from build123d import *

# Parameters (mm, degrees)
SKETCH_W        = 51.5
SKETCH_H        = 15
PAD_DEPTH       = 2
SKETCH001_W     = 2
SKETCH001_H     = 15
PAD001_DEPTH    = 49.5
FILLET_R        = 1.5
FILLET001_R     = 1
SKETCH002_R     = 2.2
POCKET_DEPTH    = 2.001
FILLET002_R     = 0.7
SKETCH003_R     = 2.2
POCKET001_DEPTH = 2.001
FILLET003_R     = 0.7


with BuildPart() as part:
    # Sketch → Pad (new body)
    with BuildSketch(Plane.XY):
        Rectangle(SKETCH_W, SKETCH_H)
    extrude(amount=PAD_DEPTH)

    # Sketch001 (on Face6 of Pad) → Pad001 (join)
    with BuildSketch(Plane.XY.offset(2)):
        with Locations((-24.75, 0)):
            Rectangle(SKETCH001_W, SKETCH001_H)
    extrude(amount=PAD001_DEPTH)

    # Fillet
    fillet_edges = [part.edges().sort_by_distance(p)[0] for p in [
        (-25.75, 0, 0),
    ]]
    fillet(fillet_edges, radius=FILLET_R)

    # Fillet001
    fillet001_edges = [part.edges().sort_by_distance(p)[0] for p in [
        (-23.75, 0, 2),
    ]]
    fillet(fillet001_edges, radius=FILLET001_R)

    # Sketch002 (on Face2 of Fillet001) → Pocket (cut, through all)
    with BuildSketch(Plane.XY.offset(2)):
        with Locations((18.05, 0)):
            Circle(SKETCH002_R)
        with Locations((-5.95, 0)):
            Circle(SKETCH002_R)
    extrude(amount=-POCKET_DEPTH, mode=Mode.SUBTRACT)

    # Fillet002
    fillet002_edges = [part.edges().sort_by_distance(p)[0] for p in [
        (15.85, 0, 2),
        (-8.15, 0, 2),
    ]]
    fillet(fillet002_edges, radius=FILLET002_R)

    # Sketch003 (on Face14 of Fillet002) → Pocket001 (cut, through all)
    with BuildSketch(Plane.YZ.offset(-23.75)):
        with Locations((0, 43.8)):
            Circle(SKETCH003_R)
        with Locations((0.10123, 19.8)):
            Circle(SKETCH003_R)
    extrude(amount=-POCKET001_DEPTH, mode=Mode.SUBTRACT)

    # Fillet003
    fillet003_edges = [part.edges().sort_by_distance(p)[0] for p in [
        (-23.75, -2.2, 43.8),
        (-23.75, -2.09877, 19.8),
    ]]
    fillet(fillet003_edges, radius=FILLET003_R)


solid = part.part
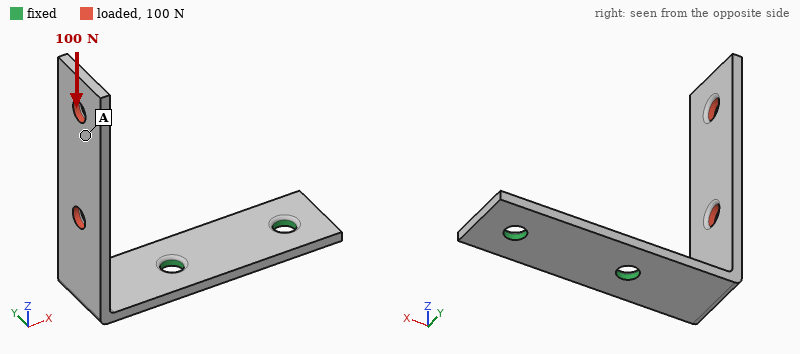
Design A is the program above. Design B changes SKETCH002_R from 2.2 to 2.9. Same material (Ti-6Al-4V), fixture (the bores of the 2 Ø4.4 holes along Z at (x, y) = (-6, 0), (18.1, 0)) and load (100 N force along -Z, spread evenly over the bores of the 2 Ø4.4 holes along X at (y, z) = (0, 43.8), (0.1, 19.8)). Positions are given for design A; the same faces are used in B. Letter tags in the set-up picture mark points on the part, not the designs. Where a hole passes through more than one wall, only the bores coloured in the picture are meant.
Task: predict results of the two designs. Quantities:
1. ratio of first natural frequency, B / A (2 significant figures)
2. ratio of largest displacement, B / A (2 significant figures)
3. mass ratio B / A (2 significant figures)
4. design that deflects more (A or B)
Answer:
1.0
0.91
0.98
A
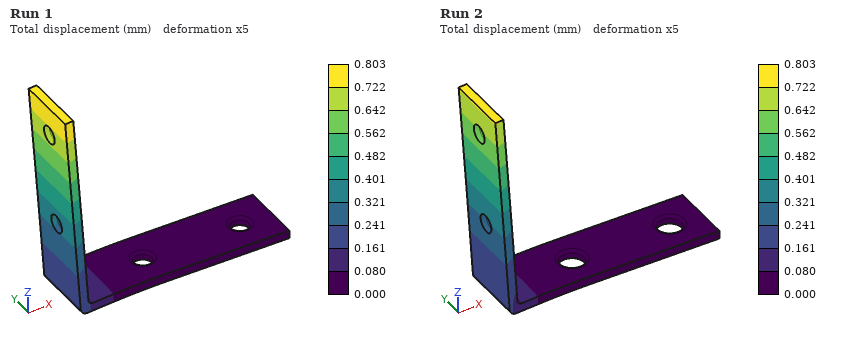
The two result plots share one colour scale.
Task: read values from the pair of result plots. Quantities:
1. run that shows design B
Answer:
Run 2
